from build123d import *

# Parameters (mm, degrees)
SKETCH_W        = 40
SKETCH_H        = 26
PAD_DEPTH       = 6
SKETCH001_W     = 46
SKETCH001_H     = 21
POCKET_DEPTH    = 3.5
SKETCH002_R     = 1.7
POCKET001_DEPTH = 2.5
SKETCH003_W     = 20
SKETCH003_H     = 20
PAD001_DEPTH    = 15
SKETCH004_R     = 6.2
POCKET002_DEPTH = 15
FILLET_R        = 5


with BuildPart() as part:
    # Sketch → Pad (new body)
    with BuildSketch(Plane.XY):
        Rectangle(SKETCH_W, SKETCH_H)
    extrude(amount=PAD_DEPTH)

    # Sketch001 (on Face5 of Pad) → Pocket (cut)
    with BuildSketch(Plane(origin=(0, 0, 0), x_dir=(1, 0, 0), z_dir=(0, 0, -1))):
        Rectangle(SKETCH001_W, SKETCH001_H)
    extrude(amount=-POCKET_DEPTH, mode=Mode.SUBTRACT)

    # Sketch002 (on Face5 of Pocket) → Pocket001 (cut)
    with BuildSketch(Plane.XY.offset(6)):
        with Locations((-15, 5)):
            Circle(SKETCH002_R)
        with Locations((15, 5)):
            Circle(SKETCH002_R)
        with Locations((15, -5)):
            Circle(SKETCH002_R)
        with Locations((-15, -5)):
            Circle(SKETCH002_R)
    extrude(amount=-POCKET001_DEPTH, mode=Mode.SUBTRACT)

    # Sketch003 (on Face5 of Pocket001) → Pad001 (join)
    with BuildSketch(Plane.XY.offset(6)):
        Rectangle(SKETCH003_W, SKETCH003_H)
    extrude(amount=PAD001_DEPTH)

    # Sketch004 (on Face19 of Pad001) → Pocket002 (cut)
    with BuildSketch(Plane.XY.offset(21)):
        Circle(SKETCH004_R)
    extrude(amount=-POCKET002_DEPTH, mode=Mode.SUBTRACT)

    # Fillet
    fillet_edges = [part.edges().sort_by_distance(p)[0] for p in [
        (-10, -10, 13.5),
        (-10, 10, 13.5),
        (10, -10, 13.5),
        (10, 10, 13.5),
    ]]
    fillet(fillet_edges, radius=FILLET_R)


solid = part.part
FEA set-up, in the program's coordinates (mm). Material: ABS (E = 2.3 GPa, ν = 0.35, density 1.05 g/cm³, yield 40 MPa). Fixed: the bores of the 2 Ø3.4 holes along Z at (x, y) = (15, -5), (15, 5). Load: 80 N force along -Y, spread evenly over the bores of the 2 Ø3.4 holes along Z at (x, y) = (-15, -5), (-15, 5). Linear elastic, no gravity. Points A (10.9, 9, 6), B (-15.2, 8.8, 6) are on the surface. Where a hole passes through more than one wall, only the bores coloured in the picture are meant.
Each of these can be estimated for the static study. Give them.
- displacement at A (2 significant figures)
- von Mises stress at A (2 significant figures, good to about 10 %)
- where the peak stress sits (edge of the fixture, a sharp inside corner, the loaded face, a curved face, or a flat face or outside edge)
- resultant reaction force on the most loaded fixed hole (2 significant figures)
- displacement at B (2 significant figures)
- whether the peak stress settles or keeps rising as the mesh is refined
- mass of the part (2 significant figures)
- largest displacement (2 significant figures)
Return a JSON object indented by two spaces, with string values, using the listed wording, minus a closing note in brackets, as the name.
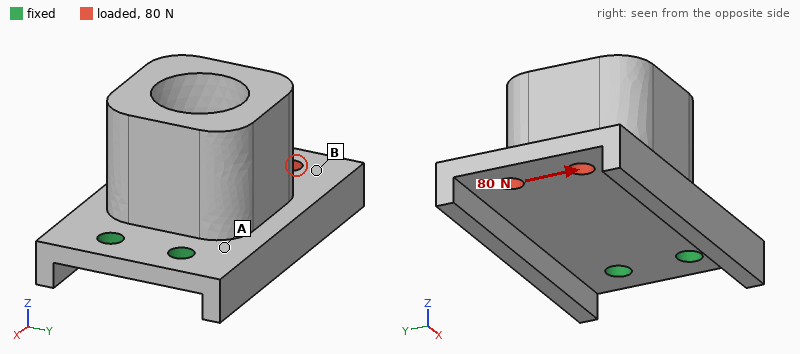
{
  "displacement at A": "0.037 mm",
  "von Mises stress at A": "5.3 MPa",
  "where the peak stress sits": "edge of the fixture",
  "resultant reaction force on the most loaded fixed hole": "190 N",
  "displacement at B": "0.19 mm",
  "whether the peak stress settles or keeps rising as the mesh is refined": "keeps rising",
  "mass of the part": "7.4 g",
  "largest displacement": "0.24 mm"
}
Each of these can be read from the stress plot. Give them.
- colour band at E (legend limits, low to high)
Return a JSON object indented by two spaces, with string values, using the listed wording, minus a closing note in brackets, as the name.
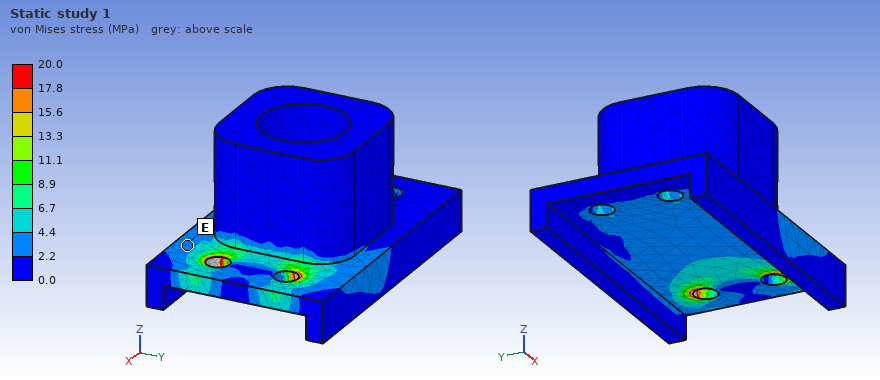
{
  "colour band at E": "2.2 to 4.4 MPa"
}
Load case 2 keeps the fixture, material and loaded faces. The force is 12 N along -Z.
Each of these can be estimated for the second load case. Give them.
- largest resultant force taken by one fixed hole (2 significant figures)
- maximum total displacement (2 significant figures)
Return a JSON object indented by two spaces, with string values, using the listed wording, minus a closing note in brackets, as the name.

{
  "largest resultant force taken by one fixed hole": "7.0 N",
  "maximum total displacement": "0.54 mm"
}
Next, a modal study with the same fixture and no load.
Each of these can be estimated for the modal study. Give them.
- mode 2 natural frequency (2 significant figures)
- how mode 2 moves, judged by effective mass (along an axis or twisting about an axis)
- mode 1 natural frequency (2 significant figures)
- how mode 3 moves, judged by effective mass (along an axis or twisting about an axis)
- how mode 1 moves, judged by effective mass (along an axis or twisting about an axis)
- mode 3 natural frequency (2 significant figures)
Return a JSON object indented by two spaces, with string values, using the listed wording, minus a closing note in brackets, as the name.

{
  "mode 2 natural frequency": "1600 Hz",
  "how mode 2 moves, judged by effective mass": "along Y",
  "mode 1 natural frequency": "500 Hz",
  "how mode 3 moves, judged by effective mass": "along Y",
  "how mode 1 moves, judged by effective mass": "along Z",
  "mode 3 natural frequency": "2200 Hz"
}
